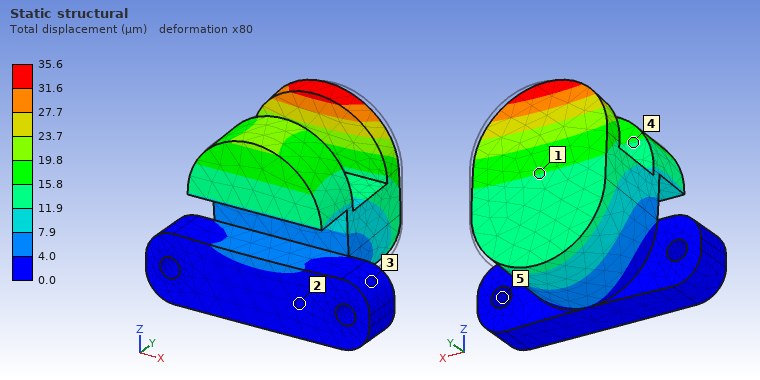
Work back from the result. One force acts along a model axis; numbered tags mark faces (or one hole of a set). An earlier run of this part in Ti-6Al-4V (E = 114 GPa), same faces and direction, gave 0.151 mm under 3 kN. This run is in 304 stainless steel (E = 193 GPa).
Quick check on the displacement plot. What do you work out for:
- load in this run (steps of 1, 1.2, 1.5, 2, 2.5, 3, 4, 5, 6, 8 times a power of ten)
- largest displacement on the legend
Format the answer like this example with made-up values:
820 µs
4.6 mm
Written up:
1.2 kN
35.6 µm
